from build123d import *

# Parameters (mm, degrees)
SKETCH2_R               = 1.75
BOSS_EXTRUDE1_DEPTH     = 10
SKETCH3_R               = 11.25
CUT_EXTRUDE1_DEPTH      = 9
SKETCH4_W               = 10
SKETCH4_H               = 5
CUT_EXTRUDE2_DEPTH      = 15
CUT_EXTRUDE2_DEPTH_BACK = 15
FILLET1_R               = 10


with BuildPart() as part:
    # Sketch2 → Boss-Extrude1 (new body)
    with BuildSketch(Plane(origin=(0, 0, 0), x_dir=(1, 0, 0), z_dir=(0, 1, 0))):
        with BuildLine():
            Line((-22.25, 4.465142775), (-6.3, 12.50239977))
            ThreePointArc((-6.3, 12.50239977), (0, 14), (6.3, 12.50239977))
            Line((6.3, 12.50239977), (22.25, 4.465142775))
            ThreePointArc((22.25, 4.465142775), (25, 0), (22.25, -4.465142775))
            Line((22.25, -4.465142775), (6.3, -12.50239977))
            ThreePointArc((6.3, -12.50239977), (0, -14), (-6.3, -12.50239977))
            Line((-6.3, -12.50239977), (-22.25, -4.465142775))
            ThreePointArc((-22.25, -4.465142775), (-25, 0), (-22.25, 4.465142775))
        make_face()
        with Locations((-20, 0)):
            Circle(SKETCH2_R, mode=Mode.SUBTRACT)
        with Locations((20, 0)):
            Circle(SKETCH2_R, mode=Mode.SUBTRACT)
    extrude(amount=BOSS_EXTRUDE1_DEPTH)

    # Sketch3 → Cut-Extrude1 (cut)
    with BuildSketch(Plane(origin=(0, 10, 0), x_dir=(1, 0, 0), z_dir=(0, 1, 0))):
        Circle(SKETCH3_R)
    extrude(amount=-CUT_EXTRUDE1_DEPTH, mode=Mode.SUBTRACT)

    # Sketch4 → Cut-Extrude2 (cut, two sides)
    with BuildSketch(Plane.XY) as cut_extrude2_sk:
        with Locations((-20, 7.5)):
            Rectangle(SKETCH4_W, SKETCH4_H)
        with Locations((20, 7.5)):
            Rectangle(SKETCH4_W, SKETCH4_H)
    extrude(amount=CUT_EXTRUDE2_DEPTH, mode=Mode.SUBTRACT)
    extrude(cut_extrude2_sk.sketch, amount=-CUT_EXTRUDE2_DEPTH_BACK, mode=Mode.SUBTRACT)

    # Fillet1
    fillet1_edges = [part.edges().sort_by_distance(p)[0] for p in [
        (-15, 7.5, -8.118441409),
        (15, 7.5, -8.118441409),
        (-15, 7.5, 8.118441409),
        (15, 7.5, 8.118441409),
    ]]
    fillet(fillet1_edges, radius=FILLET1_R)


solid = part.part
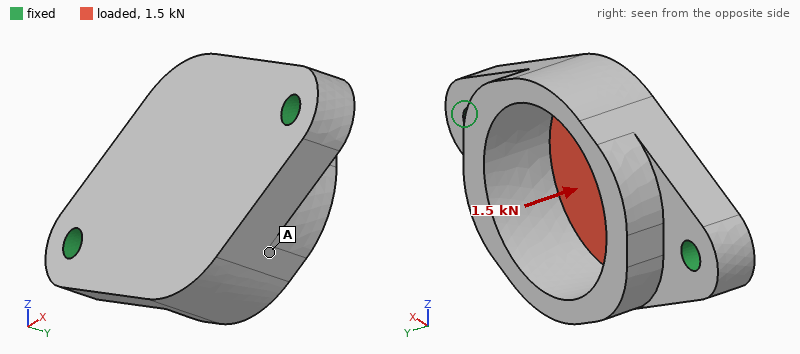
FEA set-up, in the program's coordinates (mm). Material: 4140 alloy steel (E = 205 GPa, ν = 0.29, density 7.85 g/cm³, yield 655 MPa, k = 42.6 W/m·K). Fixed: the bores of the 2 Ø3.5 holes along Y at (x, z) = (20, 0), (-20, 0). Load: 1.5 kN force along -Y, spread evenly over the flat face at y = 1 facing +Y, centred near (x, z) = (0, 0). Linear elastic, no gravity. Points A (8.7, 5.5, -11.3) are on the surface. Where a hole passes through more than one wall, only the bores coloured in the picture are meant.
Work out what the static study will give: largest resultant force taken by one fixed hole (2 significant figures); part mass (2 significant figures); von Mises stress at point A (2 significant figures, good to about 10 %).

770 N
34 g
46 MPa
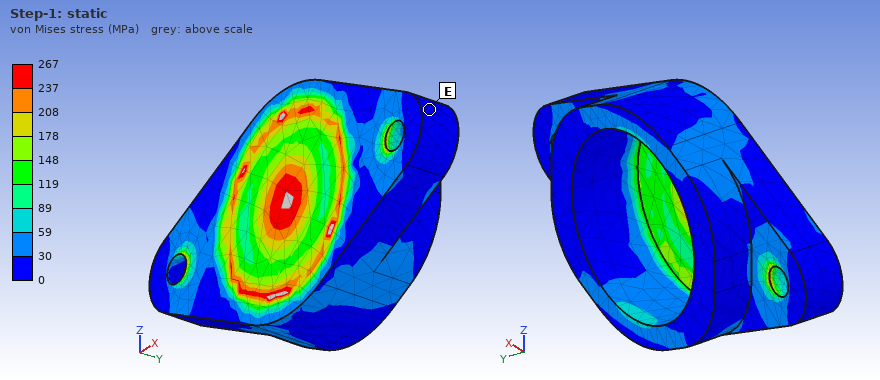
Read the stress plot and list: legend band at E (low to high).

0 to 30 MPa
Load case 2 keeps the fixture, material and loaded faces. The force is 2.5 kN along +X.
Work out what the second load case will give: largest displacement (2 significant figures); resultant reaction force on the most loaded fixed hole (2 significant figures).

3.6 µm
1.3 kN
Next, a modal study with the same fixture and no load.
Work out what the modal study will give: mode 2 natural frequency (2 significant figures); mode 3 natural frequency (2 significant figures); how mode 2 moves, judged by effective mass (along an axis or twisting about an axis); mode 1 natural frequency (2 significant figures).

13 kHz
19 kHz
along Y
11 kHz
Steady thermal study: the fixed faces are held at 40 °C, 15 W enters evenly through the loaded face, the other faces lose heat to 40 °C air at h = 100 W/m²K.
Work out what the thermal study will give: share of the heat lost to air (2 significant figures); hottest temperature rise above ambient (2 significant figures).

33 %
47 K
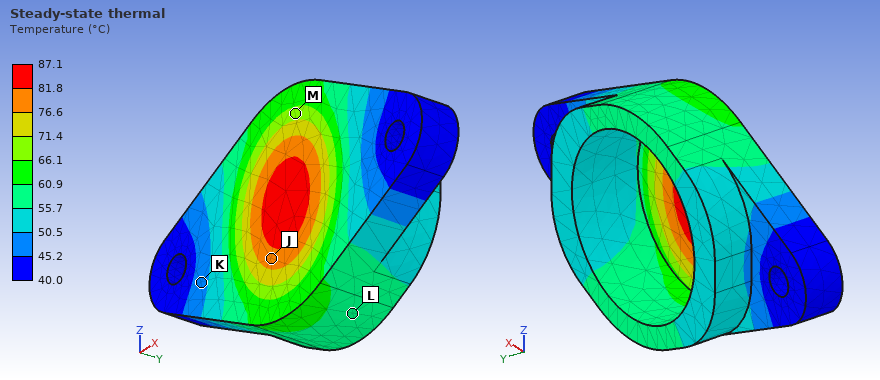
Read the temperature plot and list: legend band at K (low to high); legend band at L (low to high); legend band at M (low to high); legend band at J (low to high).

45.2 to 50.5 °C
55.7 to 60.9 °C
66.1 to 71.4 °C
76.6 to 81.8 °C
